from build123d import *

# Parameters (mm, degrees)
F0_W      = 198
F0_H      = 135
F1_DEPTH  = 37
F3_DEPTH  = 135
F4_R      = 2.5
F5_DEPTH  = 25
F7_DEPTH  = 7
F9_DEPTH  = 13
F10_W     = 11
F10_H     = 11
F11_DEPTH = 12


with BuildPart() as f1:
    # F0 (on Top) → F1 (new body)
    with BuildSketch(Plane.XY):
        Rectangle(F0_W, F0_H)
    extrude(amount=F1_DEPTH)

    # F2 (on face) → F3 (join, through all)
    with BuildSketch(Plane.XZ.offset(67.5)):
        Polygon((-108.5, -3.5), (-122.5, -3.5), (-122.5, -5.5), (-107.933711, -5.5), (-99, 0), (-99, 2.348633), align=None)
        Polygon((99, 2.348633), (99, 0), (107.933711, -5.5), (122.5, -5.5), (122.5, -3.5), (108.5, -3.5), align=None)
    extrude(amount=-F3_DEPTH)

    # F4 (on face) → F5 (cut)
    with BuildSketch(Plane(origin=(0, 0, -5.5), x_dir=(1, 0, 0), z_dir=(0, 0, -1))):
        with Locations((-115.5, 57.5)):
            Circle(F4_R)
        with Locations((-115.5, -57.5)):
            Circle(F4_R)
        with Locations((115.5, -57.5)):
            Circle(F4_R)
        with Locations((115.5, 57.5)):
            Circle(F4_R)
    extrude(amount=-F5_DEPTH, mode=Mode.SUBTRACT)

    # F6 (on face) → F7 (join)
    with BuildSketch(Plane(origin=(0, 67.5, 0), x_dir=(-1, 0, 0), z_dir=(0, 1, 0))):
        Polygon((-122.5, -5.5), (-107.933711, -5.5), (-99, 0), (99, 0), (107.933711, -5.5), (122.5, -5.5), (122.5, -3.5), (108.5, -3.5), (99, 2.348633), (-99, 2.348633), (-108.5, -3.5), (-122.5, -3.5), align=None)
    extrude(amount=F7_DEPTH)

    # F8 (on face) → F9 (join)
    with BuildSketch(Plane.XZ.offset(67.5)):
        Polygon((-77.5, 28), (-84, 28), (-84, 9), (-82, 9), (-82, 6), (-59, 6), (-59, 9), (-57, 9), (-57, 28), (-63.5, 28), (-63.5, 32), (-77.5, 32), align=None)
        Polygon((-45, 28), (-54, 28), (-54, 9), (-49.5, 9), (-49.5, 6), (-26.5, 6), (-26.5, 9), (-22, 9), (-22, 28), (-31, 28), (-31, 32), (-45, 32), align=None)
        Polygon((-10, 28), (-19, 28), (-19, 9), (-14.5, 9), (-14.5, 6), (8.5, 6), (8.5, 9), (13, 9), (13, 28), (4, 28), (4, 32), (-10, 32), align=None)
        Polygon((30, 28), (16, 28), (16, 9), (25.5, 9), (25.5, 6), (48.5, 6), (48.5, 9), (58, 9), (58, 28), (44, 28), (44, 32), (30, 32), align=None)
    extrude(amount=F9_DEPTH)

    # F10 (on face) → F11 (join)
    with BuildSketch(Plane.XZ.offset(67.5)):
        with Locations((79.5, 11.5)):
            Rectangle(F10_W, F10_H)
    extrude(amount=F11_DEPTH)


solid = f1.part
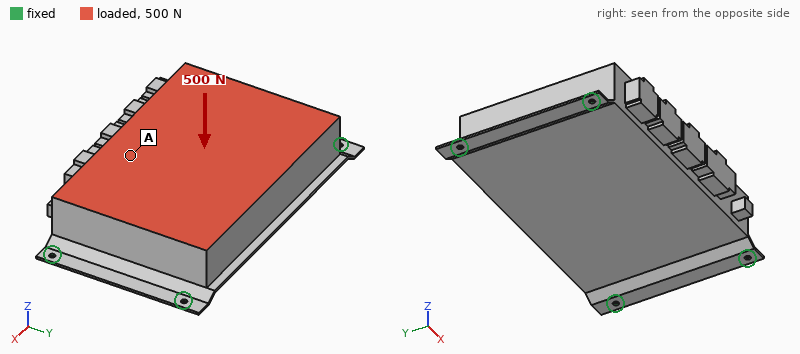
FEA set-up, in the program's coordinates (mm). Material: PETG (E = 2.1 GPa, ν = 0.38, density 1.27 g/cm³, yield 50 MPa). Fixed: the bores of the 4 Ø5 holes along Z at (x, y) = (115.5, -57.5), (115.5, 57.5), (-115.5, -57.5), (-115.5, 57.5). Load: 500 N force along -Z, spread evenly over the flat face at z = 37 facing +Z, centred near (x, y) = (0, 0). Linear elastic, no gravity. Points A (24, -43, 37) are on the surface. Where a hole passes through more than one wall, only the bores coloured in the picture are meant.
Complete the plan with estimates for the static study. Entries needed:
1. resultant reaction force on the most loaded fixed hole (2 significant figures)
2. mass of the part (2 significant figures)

270 N
1.3 kg
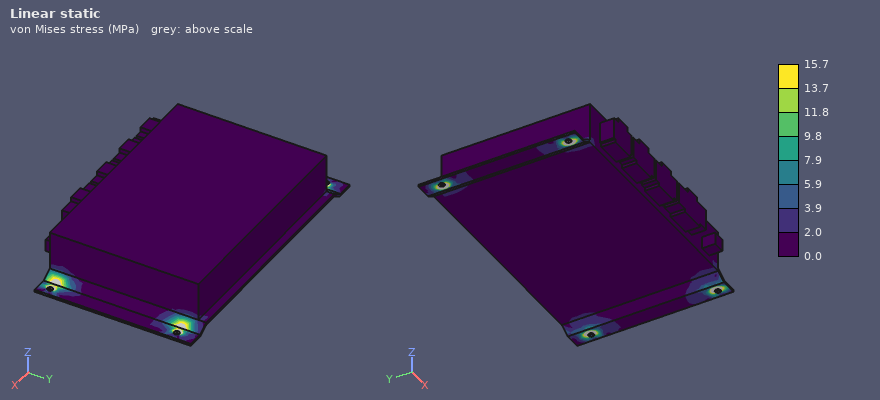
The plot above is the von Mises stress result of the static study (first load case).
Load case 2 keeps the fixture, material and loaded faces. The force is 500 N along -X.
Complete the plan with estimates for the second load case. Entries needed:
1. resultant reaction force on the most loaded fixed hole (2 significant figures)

140 N
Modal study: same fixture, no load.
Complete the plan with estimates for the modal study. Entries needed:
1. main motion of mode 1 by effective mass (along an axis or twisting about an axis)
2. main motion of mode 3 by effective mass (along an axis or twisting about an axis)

along Z
along Y
